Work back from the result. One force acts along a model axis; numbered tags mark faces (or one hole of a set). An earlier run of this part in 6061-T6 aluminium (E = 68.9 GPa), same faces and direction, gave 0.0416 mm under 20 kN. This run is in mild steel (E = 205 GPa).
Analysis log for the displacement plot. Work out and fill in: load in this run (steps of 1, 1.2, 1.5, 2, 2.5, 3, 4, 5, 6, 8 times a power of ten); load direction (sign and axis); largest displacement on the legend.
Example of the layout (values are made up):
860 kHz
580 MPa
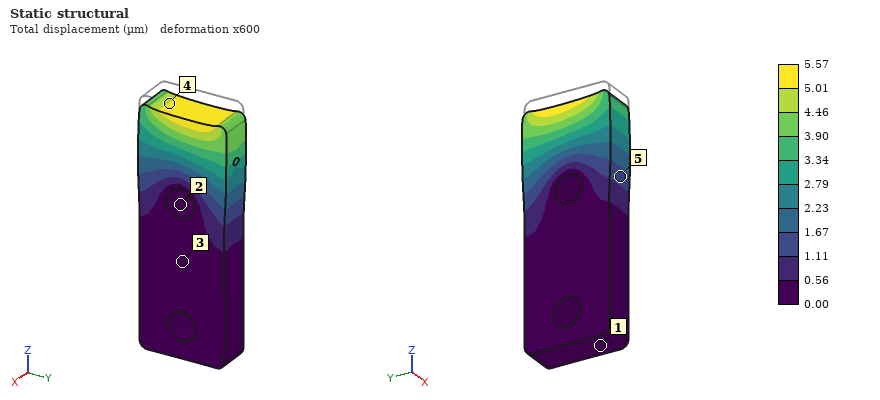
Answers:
8 kN
-Z
5.57 µm
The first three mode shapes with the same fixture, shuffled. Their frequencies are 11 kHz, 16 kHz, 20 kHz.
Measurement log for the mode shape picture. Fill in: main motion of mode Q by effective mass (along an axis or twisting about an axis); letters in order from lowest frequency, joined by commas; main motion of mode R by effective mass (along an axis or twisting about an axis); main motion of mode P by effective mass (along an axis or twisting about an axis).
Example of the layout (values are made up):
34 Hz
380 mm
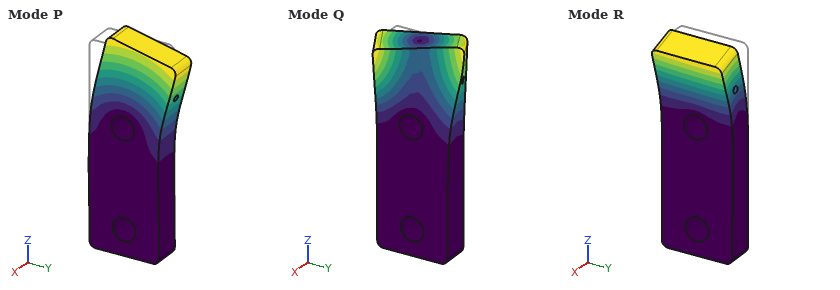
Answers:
twisting about Z
R, P, Q
along X
along Y
